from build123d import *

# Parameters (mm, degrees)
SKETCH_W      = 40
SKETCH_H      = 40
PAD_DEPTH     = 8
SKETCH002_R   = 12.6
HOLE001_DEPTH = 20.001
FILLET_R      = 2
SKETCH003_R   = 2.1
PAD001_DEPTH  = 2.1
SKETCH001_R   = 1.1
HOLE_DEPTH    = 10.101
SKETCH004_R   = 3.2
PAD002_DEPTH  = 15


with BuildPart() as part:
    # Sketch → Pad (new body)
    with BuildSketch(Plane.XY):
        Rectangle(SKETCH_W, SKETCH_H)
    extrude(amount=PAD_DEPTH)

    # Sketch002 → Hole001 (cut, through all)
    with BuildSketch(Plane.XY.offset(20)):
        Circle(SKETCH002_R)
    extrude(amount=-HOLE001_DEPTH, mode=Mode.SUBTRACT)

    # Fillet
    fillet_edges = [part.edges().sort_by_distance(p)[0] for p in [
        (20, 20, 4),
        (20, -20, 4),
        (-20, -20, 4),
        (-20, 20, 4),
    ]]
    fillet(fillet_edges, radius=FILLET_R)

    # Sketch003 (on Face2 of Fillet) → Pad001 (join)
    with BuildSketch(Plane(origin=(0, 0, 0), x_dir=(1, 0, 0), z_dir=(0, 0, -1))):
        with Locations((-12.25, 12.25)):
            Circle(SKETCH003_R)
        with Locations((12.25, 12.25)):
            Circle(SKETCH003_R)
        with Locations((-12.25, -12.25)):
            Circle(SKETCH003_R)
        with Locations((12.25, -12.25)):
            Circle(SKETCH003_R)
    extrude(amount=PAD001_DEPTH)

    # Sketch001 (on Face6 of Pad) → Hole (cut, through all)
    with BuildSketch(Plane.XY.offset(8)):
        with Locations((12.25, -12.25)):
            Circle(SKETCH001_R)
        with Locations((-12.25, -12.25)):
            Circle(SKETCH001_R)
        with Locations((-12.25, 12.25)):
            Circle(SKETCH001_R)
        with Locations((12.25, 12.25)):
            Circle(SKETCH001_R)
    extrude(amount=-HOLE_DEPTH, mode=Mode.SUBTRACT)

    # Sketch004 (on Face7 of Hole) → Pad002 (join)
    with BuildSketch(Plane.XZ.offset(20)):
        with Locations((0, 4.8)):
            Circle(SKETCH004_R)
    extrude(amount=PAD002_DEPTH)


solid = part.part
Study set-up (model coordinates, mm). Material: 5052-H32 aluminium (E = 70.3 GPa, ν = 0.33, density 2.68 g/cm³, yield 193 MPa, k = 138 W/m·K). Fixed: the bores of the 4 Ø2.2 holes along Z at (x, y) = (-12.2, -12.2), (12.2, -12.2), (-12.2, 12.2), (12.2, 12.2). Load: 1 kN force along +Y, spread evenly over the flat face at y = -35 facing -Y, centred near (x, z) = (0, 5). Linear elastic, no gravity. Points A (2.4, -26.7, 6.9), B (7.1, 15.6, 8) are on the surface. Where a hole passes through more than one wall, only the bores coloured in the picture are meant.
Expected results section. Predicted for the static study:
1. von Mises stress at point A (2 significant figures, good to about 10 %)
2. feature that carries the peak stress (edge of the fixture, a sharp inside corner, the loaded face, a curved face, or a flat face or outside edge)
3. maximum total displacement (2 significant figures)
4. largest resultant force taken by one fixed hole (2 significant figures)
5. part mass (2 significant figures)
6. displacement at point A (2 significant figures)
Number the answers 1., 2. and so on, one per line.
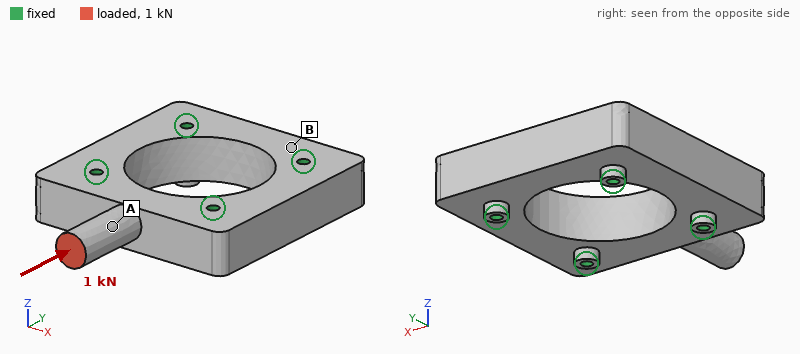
1. 31 MPa
2. a flat face or outside edge
3. 14 µm
4. 680 N
5. 25 g
6. 9.8 µm
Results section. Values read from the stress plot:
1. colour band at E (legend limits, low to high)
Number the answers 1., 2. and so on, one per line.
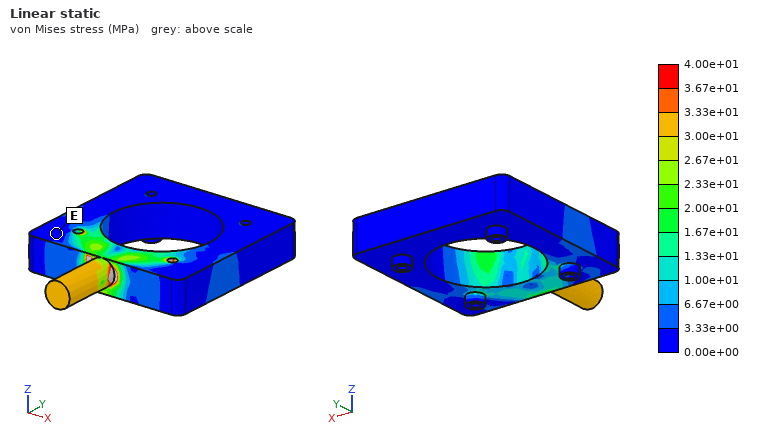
1. 0.00e+00 to 3.33e+00 MPa
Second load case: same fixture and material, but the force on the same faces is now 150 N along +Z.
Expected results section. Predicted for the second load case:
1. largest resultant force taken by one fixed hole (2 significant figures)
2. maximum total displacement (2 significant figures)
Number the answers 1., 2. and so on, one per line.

1. 88 N
2. 62 µm
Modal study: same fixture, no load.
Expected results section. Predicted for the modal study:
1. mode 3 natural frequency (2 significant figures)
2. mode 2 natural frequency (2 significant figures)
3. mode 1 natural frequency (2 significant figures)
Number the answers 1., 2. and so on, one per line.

1. 35 kHz
2. 15 kHz
3. 12 kHz
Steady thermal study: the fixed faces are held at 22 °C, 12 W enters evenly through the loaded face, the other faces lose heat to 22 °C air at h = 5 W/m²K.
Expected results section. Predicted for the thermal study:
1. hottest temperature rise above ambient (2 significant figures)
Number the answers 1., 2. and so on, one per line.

1. 52 K
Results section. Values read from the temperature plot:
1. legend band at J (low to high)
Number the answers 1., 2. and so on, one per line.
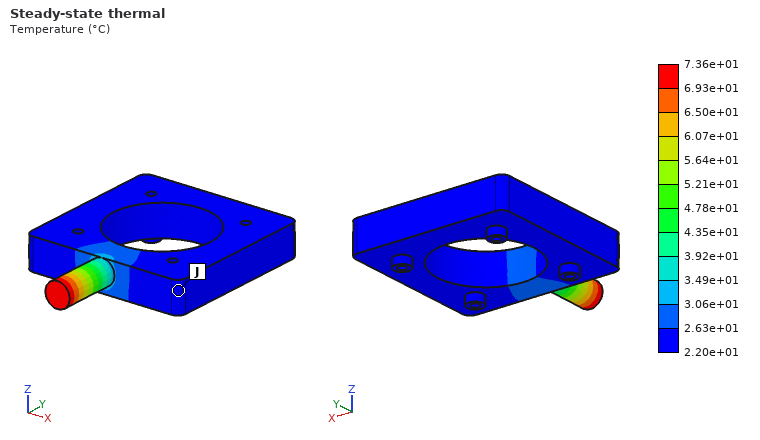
1. 2.20e+01 to 2.63e+01 °C
